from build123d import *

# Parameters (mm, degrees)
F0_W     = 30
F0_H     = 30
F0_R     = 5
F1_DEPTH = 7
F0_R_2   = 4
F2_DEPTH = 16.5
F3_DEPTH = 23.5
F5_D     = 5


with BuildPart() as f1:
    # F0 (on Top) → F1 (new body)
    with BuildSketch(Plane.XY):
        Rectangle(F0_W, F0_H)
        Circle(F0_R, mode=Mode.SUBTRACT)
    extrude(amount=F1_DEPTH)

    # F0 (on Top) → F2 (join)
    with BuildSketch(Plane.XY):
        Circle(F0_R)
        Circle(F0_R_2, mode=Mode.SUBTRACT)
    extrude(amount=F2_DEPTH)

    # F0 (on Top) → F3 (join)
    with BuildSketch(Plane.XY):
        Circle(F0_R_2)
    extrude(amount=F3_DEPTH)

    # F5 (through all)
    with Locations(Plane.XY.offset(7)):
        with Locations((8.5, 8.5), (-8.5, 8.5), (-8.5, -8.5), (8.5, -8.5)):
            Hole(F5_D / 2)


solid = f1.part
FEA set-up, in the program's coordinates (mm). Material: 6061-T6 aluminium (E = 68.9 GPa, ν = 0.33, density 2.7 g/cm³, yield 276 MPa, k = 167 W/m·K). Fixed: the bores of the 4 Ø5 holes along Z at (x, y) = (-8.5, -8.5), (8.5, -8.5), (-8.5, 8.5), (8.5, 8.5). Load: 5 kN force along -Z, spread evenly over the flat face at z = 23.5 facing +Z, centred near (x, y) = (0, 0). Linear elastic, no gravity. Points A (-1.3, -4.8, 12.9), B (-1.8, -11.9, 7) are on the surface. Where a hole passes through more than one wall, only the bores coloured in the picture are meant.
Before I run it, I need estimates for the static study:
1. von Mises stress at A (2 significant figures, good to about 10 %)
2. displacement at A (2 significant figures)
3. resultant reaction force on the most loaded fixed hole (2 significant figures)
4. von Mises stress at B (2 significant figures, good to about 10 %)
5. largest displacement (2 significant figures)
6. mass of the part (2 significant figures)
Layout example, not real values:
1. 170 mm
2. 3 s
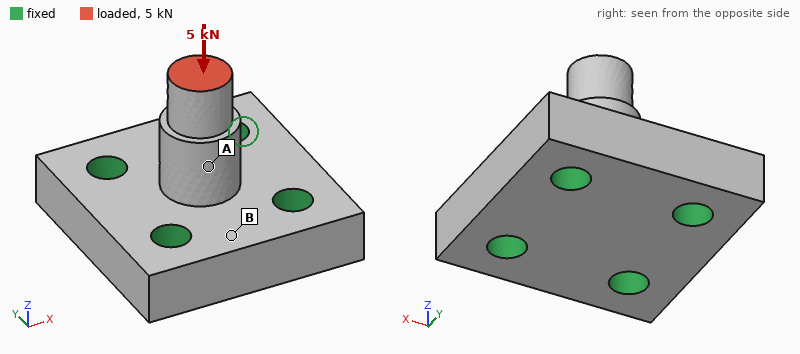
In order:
1. 57 MPa
2. 13 µm
3. 1.3 kN
4. 9.3 MPa
5. 28 µm
6. 18 g
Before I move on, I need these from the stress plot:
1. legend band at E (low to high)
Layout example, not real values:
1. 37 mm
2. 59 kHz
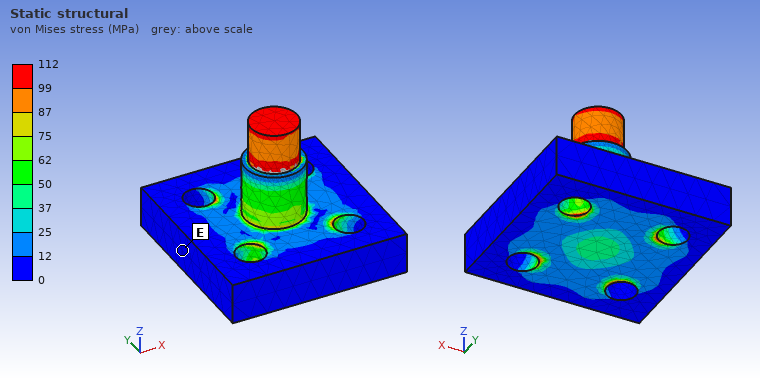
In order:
1. 0 to 12 MPa
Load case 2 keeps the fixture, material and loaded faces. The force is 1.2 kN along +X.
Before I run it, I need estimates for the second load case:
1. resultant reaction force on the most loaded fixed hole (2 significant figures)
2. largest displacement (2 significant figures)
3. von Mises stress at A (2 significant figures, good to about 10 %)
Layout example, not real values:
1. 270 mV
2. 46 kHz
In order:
1. 870 N
2. 0.11 mm
3. 43 MPa
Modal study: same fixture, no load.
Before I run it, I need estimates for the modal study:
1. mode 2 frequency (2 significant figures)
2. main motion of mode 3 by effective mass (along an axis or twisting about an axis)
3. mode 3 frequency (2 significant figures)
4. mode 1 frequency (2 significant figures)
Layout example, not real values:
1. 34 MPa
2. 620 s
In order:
1. 21 kHz
2. along Z
3. 49 kHz
4. 20 kHz
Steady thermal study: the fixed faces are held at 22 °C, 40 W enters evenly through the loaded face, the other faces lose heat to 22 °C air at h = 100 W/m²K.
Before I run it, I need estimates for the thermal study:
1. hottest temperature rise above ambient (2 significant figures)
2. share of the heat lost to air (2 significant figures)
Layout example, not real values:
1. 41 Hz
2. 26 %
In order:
1. 72 K
2. 5.0 %
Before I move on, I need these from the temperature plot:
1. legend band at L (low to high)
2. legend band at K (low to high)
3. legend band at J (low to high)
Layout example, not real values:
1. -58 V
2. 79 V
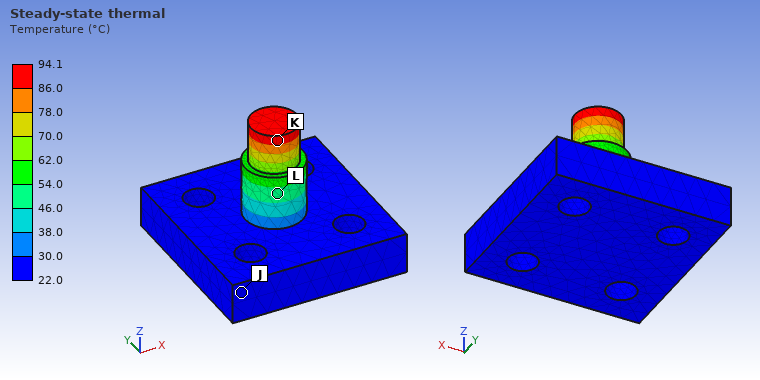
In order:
1. 46.0 to 54.0 °C
2. 86.0 to 94.1 °C
3. 22.0 to 30.0 °C
